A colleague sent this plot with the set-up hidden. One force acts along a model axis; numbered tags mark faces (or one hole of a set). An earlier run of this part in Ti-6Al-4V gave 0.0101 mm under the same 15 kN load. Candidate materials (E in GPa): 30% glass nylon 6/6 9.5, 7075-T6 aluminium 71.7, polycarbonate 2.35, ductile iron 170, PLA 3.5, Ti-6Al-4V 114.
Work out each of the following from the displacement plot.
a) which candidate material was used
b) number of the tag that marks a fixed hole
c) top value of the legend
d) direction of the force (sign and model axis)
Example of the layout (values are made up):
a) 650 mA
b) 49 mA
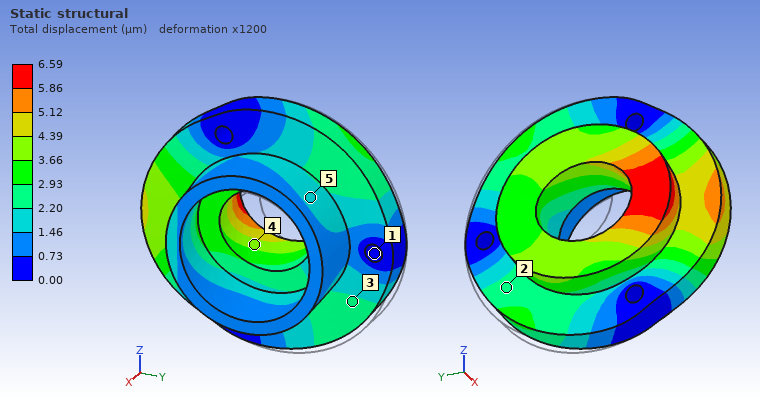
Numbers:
a) ductile iron
b) 1
c) 6.59 µm
d) -Y
